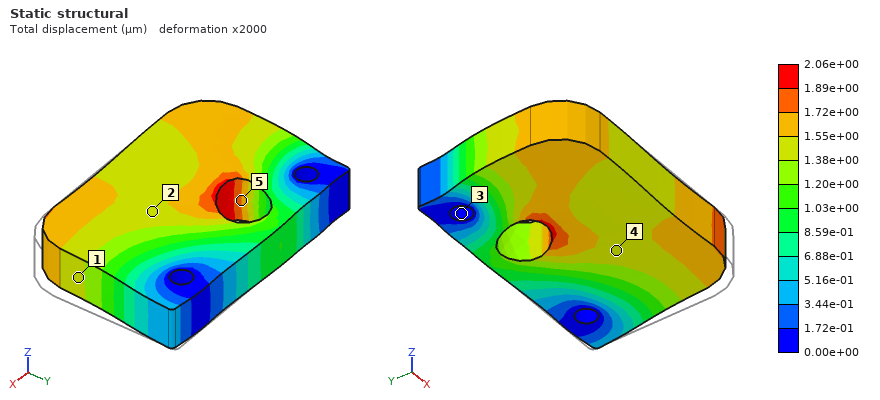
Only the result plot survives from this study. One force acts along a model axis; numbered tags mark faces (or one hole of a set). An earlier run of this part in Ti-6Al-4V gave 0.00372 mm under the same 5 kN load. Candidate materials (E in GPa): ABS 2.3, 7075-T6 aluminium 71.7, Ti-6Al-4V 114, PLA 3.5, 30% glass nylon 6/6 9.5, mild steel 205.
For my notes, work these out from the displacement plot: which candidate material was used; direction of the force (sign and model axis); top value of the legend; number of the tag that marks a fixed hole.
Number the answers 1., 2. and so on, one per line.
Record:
1. mild steel
2. -X
3. 2.06e+00 µm
4. 3
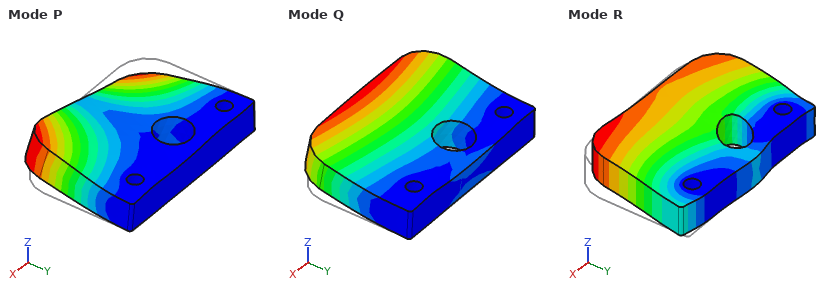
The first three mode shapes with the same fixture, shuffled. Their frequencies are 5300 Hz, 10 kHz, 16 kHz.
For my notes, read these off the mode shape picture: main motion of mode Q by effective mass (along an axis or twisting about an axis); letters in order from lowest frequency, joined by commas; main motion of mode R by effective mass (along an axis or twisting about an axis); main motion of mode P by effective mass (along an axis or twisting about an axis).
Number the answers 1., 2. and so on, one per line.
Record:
1. along Z
2. Q, P, R
3. along X
4. twisting about Y
